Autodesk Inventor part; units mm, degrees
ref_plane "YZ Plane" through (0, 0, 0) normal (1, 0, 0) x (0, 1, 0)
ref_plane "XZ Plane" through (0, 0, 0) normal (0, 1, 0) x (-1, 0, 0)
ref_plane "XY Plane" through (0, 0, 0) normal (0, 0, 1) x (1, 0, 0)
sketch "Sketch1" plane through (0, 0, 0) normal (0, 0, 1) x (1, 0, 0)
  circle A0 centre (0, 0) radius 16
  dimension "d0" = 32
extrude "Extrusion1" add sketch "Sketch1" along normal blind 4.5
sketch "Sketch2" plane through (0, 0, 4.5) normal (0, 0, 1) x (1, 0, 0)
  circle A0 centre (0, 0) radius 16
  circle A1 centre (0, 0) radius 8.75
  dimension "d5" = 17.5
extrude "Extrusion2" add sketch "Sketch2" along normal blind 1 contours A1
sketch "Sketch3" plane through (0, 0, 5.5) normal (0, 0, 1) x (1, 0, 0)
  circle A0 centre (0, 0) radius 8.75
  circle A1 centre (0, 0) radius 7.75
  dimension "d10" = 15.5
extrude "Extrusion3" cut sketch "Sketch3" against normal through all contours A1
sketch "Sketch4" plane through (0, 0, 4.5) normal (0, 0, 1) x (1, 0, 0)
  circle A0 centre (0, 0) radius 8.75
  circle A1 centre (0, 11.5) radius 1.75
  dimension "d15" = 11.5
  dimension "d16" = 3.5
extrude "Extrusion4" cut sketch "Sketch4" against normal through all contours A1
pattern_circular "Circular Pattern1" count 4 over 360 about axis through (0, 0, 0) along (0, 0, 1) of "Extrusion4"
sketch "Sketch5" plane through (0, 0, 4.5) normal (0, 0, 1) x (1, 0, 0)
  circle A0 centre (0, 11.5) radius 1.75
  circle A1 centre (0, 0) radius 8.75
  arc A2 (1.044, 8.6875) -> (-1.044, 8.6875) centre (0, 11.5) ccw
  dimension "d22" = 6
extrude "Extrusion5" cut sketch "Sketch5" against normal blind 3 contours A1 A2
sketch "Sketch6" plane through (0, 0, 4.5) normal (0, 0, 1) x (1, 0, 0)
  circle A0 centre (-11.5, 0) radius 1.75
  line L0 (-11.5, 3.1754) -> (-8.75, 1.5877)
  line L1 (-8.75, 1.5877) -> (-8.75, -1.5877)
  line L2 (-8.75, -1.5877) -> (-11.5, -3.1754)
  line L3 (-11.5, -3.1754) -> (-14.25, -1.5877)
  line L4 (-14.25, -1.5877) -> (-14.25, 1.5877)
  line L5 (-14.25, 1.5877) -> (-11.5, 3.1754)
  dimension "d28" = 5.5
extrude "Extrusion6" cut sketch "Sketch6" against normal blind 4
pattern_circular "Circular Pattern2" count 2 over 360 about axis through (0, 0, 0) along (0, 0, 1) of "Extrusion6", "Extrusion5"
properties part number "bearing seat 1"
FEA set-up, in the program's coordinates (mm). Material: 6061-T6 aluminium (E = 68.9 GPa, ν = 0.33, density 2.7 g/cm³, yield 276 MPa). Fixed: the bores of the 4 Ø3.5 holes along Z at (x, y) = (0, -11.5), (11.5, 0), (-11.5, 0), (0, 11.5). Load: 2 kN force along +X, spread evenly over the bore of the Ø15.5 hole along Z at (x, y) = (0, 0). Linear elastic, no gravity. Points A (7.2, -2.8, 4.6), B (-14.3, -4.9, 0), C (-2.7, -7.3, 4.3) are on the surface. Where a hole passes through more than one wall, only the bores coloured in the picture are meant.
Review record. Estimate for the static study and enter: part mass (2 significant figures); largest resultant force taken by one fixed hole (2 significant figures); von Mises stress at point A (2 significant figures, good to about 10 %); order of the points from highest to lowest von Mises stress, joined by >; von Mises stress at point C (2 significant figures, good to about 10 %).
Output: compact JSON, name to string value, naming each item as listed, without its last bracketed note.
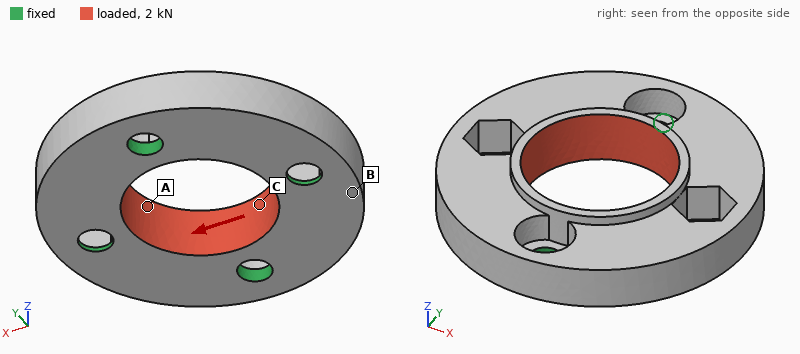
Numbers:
{"part mass": "6.5 g", "largest resultant force taken by one fixed hole": "700 N", "von Mises stress at point A": "48 MPa", "order of the points from highest to lowest von Mises stress, joined by >": "A > C > B", "von Mises stress at point C": "23 MPa"}
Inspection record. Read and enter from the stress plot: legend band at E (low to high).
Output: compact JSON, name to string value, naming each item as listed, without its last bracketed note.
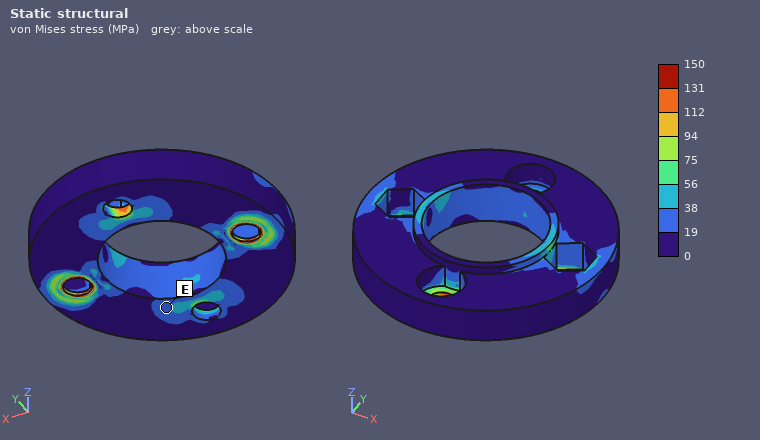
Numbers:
{"legend band at E": "19 to 38 MPa"}
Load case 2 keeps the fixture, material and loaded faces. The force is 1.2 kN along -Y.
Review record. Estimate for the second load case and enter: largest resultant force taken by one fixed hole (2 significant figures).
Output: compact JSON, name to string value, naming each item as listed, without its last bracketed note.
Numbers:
{"largest resultant force taken by one fixed hole": "370 N"}
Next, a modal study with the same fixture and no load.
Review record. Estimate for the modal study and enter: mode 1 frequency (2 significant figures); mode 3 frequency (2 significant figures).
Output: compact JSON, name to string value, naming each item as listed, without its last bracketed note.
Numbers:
{"mode 1 frequency": "20 kHz", "mode 3 frequency": "26 kHz"}
